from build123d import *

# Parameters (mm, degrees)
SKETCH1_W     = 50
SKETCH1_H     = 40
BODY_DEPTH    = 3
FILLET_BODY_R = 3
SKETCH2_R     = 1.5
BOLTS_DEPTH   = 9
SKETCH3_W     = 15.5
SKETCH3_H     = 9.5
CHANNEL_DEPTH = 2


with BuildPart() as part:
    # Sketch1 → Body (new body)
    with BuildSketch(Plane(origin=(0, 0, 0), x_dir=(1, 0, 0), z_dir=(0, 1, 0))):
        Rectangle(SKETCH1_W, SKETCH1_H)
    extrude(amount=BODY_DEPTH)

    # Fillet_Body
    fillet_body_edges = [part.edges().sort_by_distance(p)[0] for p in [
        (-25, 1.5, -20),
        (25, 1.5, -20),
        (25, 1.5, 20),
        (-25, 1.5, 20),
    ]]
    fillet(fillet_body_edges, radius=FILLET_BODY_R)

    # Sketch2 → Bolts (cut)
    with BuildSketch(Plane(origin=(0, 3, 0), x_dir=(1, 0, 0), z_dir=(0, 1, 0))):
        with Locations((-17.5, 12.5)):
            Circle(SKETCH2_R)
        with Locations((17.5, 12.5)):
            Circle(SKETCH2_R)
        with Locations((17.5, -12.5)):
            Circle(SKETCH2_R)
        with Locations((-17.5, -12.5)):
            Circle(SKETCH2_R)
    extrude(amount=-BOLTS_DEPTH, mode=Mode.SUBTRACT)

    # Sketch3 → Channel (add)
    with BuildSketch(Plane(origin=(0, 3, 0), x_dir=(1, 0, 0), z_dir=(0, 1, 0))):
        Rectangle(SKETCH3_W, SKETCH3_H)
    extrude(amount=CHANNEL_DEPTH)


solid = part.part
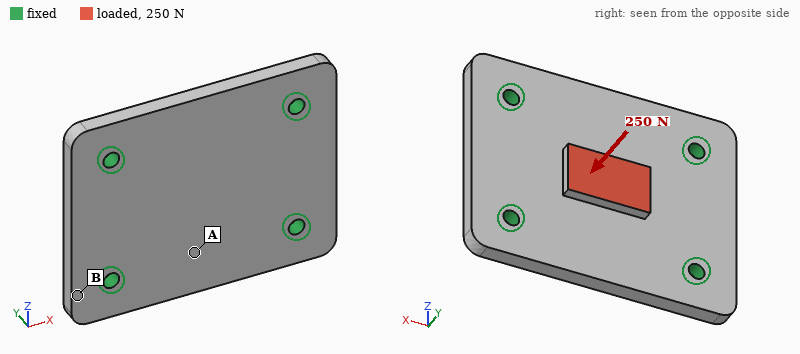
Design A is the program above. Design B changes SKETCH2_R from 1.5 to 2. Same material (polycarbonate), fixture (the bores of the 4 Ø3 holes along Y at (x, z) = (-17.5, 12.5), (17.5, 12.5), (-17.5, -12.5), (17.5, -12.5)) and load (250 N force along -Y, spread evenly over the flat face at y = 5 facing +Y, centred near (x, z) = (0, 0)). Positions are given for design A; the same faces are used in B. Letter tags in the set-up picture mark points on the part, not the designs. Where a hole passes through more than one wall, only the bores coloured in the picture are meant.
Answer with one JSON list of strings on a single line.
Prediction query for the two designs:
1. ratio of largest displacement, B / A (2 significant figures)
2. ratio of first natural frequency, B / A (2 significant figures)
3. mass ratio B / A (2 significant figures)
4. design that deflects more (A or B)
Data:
["0.90", "1.1", "0.99", "A"]
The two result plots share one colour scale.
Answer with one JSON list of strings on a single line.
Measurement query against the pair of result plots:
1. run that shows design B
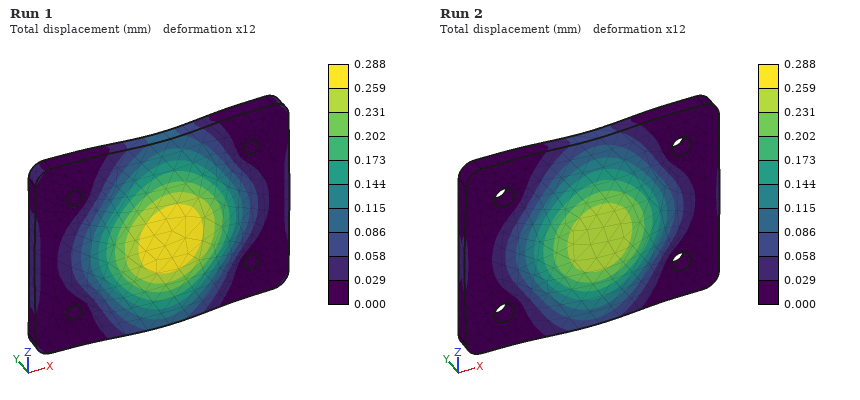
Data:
["Run 2"]
